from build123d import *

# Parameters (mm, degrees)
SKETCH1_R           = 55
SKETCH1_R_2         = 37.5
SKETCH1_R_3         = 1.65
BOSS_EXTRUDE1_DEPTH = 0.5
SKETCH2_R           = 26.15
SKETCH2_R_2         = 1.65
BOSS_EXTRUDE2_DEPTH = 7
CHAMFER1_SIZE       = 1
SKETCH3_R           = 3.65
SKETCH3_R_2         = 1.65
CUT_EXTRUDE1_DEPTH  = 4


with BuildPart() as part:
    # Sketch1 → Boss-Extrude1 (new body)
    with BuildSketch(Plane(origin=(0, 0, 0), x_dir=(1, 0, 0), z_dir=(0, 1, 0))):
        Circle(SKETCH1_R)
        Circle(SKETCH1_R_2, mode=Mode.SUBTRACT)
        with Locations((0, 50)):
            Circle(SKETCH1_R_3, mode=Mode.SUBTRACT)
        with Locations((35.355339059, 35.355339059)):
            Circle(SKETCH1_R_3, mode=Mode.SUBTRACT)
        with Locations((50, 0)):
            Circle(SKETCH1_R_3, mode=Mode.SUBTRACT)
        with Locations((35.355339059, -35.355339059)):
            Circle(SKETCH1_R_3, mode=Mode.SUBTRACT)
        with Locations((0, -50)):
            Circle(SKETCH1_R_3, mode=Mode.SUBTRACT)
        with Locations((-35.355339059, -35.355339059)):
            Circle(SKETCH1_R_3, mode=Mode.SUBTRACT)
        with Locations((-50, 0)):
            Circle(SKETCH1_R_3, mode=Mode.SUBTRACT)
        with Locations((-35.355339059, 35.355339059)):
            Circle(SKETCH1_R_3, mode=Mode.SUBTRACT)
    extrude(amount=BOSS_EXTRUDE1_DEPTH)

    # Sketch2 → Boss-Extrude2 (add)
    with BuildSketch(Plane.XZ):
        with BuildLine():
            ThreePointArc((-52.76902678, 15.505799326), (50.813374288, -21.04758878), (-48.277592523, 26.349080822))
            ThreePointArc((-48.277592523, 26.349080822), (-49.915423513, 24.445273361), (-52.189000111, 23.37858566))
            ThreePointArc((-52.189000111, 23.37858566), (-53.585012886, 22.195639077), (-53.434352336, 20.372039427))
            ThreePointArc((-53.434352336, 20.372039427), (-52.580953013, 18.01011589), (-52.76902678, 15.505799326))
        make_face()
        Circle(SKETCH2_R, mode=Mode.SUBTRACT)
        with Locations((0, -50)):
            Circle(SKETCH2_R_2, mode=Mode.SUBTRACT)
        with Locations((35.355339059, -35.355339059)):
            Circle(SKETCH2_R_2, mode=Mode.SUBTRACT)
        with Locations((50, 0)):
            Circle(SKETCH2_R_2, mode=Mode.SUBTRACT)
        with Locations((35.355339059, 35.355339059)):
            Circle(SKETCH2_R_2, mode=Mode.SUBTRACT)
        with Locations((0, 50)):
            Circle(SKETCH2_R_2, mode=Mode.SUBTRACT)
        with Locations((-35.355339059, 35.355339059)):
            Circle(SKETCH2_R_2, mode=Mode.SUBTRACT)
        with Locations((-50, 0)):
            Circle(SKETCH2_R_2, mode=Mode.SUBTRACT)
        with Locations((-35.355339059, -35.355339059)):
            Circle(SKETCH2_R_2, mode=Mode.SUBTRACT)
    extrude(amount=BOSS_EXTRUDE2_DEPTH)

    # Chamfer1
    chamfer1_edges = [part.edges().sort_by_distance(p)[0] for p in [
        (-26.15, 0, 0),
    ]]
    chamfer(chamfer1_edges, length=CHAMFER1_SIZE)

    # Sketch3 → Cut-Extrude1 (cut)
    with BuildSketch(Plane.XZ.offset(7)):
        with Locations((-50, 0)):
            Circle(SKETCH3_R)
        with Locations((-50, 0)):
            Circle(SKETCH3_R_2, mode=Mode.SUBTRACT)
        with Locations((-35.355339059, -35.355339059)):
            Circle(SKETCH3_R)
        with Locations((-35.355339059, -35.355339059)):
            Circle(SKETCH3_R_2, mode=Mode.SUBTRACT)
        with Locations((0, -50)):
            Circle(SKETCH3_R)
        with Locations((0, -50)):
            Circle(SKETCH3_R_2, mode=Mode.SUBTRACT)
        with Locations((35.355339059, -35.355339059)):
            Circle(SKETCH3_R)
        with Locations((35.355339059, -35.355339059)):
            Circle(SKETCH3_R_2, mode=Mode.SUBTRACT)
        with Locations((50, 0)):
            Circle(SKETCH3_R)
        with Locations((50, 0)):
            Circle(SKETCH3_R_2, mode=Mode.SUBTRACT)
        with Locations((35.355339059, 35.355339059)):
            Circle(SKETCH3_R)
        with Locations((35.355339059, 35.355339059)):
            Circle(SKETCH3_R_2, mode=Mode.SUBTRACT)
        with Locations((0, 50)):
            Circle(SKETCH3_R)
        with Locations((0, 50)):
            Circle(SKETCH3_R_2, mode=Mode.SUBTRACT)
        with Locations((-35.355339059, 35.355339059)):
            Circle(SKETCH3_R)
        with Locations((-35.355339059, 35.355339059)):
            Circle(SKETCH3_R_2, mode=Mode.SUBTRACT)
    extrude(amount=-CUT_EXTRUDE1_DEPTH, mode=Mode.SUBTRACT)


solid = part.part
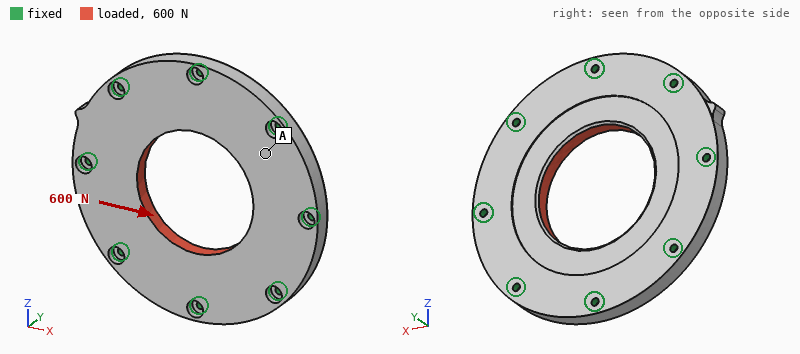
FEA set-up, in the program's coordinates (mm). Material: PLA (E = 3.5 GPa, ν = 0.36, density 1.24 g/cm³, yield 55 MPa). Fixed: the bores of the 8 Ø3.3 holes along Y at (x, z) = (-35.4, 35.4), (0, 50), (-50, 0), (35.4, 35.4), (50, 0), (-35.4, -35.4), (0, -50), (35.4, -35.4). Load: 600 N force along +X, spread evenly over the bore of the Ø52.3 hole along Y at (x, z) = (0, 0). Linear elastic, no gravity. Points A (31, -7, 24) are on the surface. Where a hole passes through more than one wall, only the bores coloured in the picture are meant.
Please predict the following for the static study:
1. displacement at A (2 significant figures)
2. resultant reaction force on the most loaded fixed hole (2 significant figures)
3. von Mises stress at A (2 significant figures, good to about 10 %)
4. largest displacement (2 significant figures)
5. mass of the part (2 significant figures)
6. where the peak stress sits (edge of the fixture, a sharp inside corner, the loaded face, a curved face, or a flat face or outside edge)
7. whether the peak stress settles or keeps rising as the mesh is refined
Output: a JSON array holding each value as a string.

["8.8 µm", "96 N", "0.56 MPa", "19 µm", "65 g", "edge of the fixture", "keeps rising"]
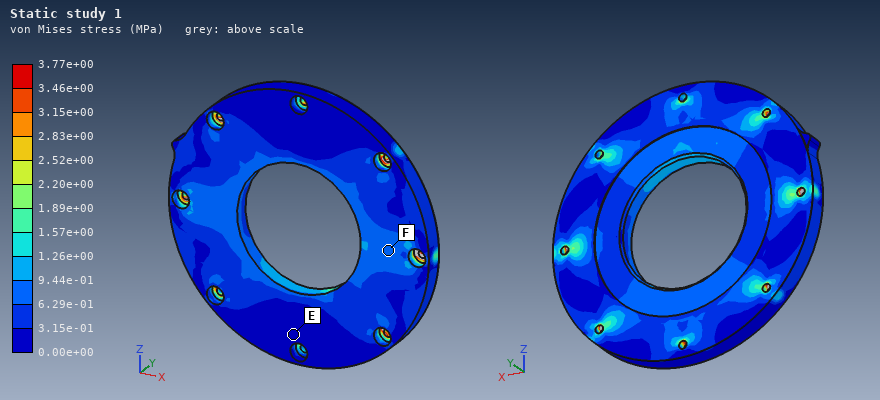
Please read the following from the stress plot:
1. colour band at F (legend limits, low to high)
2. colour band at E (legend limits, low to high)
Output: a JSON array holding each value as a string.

["6.29e-01 to 9.44e-01 MPa", "0.00e+00 to 3.15e-01 MPa"]
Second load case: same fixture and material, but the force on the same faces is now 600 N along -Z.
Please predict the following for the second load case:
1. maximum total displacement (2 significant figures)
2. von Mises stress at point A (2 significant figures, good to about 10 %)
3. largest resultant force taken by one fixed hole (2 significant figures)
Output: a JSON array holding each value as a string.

["19 µm", "0.55 MPa", "96 N"]
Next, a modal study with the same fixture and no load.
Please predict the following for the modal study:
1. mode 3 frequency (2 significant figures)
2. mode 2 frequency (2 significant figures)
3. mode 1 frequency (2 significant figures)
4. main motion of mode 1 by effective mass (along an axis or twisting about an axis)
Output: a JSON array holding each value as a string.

["2900 Hz", "2900 Hz", "2100 Hz", "along Y"]
